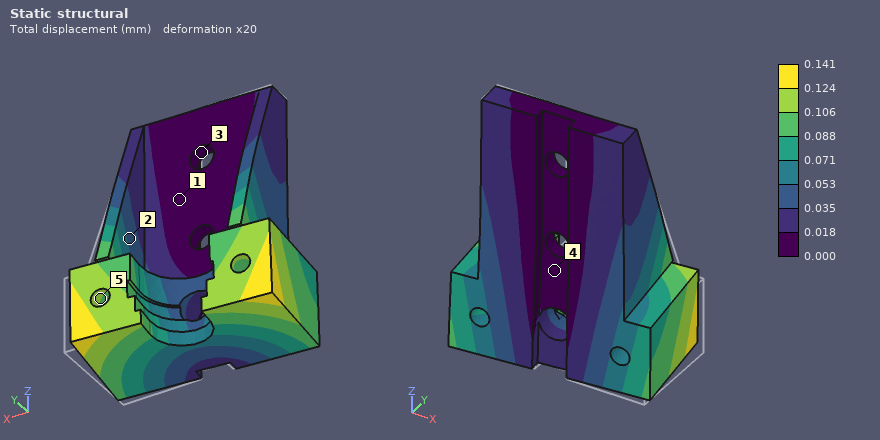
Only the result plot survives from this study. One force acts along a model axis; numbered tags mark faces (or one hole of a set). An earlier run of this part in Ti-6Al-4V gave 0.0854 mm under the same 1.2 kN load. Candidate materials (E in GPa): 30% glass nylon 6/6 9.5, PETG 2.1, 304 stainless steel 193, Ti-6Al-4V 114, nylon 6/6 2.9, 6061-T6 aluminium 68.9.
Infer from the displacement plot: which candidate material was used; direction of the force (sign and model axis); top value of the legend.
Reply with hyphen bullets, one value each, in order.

- 6061-T6 aluminium
- -X
- 0.141 mm
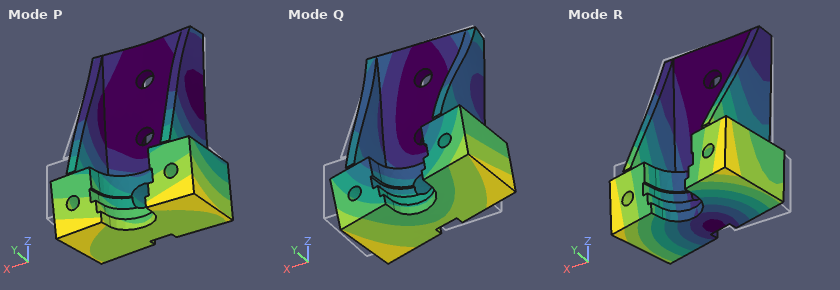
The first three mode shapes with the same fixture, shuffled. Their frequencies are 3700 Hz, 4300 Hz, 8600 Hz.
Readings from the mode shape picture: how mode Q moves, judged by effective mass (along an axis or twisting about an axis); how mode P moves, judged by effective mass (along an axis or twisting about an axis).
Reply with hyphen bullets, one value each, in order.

- along X
- along Y
